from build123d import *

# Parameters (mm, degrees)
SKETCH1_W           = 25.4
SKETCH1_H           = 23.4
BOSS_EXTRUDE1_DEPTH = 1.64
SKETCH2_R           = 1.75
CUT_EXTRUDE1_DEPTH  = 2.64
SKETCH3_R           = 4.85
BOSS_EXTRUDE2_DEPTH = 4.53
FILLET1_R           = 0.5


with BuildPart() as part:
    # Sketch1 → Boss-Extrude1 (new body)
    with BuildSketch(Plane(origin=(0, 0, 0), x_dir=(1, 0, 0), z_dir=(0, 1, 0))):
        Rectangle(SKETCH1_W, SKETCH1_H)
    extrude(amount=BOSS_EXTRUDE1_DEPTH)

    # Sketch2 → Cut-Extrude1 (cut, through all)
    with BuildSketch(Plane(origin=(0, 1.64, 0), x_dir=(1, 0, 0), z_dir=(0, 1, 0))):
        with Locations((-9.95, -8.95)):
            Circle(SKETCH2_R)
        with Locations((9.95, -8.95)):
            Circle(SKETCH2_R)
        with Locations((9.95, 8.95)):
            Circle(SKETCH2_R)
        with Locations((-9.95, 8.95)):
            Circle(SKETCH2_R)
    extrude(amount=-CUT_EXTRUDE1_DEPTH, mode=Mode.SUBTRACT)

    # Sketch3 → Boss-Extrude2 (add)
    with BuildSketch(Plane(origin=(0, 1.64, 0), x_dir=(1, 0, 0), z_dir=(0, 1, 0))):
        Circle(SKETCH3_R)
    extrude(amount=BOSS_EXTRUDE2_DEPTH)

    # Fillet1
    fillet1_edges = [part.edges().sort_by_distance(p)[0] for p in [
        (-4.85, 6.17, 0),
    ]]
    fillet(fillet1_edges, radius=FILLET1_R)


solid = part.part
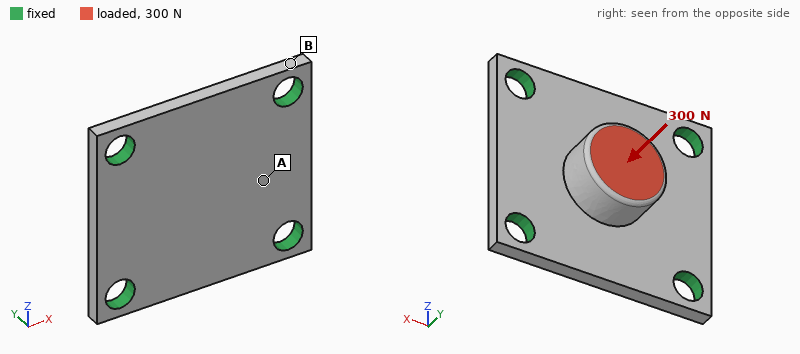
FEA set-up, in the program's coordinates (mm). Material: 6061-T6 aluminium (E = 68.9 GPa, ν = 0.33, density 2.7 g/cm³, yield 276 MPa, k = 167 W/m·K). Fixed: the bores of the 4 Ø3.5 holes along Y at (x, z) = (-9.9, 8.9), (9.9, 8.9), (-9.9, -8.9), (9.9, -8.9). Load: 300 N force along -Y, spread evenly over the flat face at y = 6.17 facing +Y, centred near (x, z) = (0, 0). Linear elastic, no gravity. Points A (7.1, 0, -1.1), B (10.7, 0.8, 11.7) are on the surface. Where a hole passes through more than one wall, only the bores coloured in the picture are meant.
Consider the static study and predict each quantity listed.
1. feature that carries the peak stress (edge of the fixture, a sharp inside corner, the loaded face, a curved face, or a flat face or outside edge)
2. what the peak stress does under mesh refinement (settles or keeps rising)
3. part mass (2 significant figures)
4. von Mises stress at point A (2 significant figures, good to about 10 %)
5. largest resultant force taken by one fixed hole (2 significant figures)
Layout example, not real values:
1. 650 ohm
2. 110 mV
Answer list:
1. edge of the fixture
2. keeps rising
3. 3.4 g
4. 25 MPa
5. 78 N
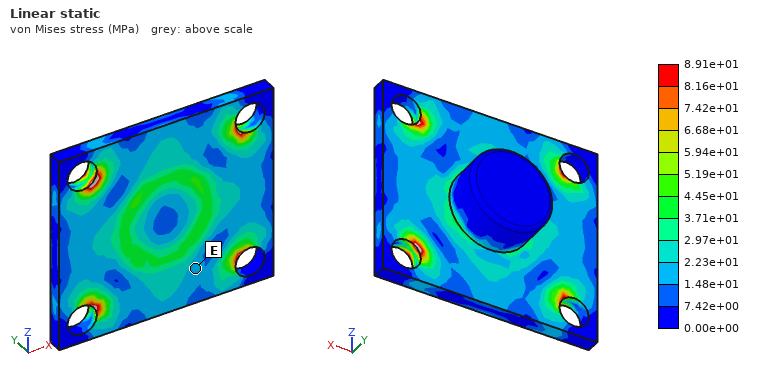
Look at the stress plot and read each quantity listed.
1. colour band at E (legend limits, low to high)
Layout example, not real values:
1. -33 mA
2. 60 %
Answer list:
1. 1.48e+01 to 2.23e+01 MPa
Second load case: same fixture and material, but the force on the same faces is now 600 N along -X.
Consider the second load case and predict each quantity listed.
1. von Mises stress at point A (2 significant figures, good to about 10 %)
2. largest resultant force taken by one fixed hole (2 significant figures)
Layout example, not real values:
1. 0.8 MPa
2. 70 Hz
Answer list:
1. 53 MPa
2. 200 N
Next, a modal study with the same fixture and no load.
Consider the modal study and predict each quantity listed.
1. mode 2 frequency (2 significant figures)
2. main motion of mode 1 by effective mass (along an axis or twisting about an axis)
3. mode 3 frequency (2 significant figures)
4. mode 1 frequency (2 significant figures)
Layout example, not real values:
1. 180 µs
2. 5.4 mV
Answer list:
1. 25 kHz
2. along Y
3. 28 kHz
4. 17 kHz
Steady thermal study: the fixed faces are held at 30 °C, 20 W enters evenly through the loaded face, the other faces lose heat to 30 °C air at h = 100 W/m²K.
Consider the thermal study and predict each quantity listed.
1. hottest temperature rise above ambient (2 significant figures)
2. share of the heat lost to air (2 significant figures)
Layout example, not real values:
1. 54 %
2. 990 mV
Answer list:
1. 25 K
2. 5.5 %
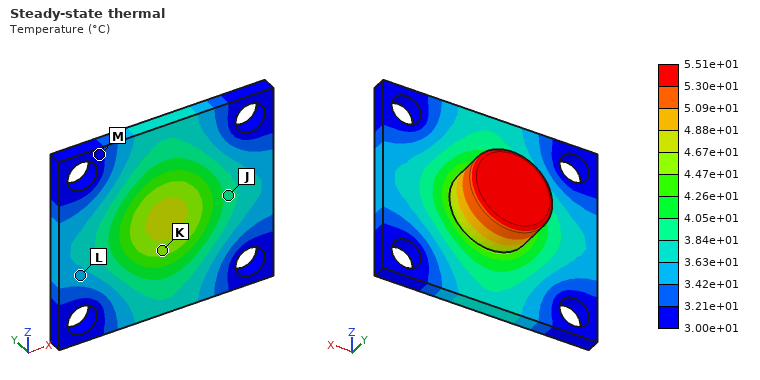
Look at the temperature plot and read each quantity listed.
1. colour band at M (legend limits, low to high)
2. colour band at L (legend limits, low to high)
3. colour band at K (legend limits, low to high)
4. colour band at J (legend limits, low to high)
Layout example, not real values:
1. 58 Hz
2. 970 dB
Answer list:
1. 3.00e+01 to 3.21e+01 °C
2. 3.42e+01 to 3.63e+01 °C
3. 4.47e+01 to 4.67e+01 °C
4. 3.84e+01 to 4.05e+01 °C
